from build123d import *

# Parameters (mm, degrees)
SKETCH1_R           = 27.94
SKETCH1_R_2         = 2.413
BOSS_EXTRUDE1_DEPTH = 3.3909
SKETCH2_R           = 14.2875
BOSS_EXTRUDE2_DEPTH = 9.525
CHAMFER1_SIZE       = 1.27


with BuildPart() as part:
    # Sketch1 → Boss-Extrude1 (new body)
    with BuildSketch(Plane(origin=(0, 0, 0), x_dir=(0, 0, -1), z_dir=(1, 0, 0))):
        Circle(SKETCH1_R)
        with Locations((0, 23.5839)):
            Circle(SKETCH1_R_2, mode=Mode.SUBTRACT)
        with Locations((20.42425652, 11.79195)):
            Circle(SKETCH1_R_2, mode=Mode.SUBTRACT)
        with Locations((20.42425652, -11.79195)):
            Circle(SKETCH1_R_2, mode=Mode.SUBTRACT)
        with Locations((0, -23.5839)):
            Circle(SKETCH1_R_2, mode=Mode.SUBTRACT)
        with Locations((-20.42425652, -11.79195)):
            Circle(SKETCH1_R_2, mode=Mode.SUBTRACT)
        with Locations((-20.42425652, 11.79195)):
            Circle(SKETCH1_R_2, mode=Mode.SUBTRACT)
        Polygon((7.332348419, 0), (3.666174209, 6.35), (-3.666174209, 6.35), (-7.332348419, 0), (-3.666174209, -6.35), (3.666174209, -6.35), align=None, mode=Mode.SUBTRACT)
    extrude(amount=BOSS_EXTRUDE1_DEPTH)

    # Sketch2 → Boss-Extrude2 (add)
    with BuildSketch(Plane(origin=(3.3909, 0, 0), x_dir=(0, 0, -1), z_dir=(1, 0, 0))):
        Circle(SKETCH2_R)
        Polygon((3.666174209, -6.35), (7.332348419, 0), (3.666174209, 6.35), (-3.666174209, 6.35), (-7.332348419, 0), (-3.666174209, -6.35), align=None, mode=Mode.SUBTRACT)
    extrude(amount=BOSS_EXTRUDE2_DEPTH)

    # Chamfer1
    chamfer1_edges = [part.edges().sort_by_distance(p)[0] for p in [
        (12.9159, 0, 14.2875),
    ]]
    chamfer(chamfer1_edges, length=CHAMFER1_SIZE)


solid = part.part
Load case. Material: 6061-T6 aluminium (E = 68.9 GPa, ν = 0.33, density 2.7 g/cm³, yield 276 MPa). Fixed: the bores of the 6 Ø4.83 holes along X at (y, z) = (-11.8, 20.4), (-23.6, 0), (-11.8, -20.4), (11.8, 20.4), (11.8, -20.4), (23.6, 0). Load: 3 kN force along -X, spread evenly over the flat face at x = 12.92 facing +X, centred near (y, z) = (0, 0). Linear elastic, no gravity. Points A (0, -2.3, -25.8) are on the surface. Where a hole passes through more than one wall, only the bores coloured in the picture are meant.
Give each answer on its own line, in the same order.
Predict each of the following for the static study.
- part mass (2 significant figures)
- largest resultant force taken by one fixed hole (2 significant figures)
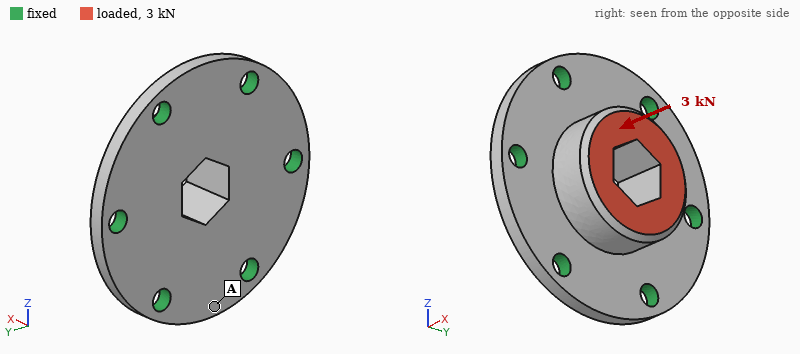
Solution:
33 g
570 N
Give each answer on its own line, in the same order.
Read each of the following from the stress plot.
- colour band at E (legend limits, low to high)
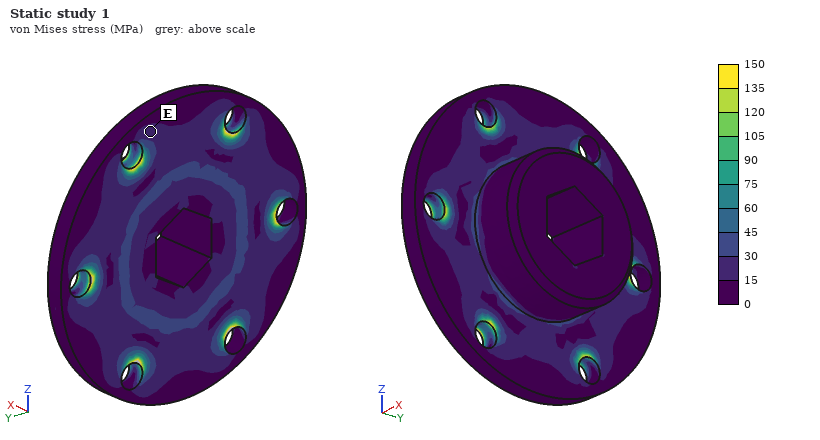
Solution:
15 to 30 MPa
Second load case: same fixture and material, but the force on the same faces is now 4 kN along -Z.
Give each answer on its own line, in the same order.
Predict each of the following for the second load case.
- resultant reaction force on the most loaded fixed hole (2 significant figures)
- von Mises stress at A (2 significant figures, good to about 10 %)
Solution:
1.1 kN
20 MPa
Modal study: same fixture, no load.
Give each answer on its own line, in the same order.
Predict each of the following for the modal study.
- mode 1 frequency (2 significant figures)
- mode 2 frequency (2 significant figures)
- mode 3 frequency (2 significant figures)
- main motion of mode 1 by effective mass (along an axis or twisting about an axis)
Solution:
15 kHz
20 kHz
20 kHz
along X
